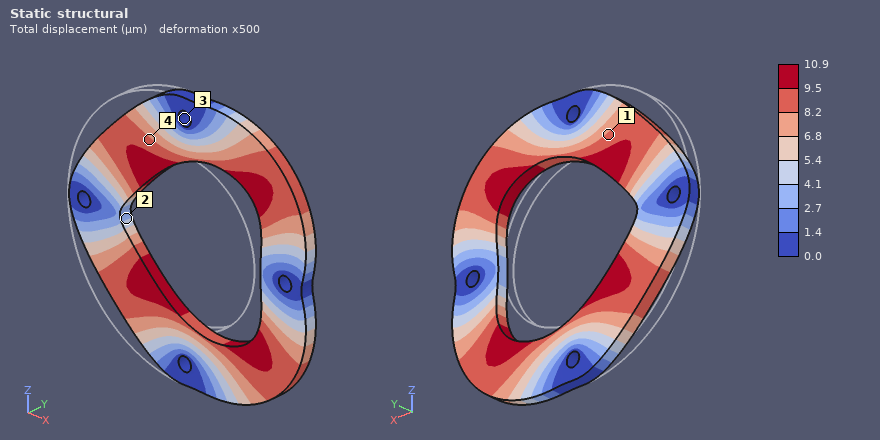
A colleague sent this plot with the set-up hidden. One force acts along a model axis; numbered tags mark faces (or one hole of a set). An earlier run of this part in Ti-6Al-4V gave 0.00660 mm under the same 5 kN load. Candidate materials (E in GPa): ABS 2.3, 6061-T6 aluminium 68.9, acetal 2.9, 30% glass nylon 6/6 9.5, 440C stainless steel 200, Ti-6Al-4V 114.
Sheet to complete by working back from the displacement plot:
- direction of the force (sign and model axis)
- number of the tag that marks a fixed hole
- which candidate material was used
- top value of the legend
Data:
+X
3
6061-T6 aluminium
10.9 µm
